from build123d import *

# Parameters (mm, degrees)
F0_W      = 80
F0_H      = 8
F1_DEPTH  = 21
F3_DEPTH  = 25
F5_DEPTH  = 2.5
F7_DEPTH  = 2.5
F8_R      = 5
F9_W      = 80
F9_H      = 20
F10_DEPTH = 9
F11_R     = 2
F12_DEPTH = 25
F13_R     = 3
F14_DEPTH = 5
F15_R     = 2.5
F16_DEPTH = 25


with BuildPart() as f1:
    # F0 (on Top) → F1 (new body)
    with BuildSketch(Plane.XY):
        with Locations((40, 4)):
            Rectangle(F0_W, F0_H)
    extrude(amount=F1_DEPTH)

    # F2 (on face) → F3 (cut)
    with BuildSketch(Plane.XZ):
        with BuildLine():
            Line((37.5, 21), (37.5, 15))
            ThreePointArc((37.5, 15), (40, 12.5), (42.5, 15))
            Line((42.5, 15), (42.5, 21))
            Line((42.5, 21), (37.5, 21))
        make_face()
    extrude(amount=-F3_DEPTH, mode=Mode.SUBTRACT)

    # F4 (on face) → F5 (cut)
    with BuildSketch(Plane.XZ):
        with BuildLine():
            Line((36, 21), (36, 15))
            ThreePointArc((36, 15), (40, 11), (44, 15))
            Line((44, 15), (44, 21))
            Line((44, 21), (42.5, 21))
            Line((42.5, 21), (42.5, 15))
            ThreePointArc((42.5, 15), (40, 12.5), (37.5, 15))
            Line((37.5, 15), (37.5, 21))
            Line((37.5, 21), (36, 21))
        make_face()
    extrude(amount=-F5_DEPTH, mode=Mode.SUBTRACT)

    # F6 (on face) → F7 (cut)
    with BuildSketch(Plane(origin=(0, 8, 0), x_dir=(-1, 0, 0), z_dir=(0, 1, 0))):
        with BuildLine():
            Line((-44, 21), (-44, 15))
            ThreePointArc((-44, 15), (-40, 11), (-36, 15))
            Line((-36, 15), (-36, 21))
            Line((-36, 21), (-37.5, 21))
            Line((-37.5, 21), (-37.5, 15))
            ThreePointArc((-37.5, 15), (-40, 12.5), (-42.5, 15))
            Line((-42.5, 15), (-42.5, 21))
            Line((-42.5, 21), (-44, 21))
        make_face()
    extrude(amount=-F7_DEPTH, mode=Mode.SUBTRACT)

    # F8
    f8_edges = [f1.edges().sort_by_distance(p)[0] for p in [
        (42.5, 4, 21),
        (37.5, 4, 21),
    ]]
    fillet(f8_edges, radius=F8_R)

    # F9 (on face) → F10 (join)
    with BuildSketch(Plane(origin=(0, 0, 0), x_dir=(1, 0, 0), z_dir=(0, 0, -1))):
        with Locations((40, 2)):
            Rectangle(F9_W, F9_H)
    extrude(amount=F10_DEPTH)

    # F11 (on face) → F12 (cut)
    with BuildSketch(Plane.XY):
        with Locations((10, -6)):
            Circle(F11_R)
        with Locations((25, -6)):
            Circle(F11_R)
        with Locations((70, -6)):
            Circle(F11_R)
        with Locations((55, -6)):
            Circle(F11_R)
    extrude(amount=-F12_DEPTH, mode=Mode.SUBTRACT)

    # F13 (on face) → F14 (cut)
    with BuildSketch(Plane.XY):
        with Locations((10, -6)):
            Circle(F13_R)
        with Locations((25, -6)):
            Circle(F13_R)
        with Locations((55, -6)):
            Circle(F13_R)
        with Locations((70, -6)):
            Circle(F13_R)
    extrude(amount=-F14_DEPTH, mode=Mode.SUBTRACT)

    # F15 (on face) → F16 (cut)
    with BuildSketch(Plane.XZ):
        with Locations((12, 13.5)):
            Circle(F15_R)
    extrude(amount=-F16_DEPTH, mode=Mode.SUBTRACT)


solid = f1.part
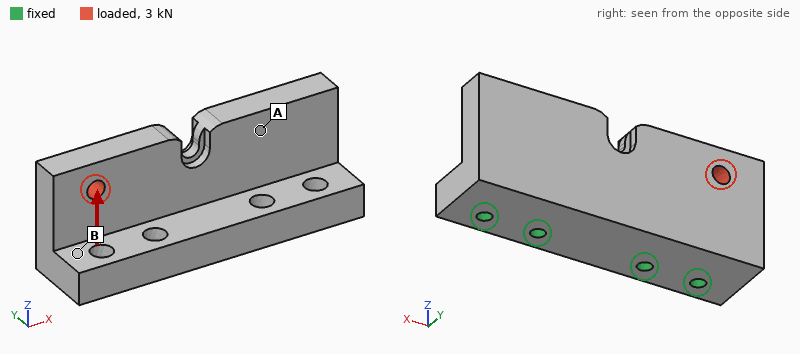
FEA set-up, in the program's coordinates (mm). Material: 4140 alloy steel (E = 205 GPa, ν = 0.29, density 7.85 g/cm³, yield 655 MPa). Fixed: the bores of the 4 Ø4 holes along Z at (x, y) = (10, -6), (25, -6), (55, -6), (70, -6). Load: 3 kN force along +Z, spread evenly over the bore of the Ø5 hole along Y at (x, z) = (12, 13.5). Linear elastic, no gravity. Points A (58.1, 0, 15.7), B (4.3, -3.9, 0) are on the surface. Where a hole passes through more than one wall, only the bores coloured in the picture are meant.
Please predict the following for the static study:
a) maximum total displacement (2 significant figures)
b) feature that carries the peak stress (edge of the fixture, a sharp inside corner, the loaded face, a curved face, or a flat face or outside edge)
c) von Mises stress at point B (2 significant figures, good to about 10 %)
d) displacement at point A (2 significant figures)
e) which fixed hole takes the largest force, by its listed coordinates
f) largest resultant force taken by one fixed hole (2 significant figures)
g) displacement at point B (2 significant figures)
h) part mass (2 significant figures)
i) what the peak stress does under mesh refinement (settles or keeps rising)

37 µm
edge of the fixture
39 MPa
11 µm
(10, -6)
2.1 kN
8.6 µm
210 g
keeps rising
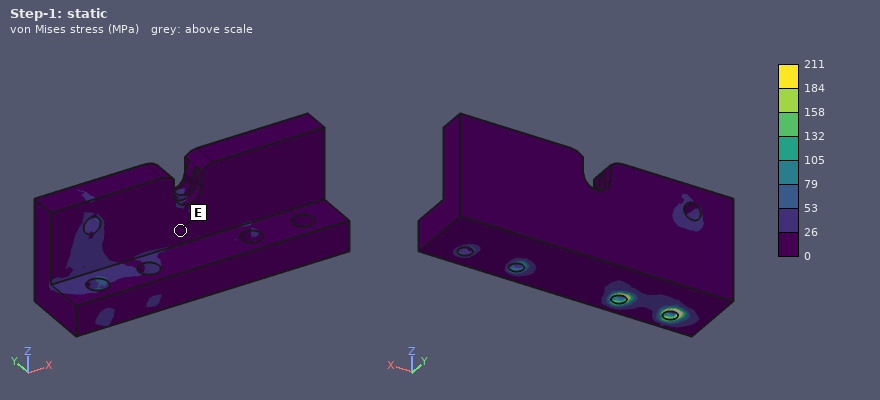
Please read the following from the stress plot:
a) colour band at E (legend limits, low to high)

0 to 26 MPa
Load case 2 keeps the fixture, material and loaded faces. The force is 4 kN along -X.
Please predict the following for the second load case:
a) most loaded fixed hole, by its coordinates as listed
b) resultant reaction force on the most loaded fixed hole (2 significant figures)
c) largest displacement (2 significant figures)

(10, -6)
2.0 kN
16 µm
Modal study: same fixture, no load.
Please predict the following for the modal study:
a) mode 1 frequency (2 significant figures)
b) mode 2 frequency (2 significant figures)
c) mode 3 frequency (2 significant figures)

4300 Hz
6700 Hz
13 kHz
